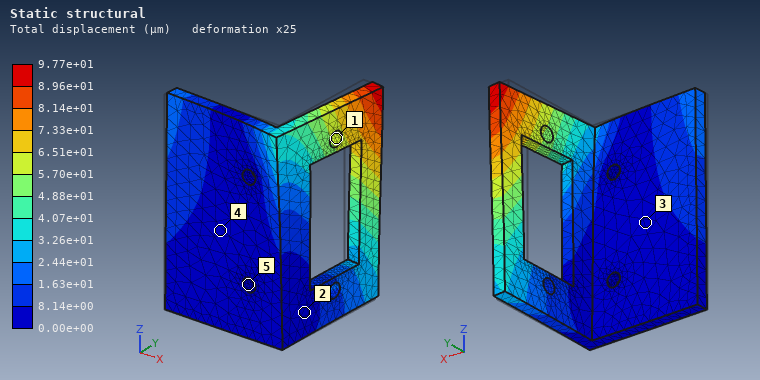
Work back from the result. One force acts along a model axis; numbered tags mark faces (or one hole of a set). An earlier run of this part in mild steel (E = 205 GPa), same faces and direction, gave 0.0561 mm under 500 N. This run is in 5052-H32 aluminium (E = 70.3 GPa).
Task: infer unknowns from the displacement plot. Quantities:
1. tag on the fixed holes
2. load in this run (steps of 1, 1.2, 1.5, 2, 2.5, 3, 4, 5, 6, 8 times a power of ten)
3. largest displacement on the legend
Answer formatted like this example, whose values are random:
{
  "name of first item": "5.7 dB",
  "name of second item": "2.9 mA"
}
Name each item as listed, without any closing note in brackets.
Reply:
{
  "tag on the fixed holes": "5",
  "load in this run": "300 N",
  "largest displacement on the legend": "9.77e+01 µm"
}
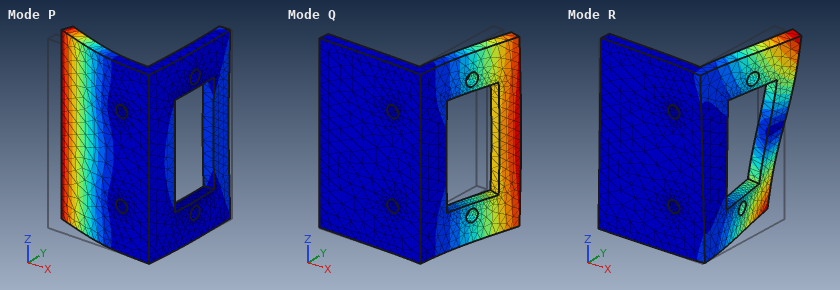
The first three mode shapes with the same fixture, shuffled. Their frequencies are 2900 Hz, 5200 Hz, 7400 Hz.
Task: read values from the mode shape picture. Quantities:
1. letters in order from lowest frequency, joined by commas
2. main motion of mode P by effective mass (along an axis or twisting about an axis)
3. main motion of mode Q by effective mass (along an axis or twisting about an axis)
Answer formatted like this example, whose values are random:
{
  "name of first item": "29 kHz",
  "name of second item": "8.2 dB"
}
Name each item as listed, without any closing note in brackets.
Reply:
{
  "letters in order from lowest frequency, joined by commas": "Q, R, P",
  "main motion of mode P by effective mass": "along Y",
  "main motion of mode Q by effective mass": "along X"
}
